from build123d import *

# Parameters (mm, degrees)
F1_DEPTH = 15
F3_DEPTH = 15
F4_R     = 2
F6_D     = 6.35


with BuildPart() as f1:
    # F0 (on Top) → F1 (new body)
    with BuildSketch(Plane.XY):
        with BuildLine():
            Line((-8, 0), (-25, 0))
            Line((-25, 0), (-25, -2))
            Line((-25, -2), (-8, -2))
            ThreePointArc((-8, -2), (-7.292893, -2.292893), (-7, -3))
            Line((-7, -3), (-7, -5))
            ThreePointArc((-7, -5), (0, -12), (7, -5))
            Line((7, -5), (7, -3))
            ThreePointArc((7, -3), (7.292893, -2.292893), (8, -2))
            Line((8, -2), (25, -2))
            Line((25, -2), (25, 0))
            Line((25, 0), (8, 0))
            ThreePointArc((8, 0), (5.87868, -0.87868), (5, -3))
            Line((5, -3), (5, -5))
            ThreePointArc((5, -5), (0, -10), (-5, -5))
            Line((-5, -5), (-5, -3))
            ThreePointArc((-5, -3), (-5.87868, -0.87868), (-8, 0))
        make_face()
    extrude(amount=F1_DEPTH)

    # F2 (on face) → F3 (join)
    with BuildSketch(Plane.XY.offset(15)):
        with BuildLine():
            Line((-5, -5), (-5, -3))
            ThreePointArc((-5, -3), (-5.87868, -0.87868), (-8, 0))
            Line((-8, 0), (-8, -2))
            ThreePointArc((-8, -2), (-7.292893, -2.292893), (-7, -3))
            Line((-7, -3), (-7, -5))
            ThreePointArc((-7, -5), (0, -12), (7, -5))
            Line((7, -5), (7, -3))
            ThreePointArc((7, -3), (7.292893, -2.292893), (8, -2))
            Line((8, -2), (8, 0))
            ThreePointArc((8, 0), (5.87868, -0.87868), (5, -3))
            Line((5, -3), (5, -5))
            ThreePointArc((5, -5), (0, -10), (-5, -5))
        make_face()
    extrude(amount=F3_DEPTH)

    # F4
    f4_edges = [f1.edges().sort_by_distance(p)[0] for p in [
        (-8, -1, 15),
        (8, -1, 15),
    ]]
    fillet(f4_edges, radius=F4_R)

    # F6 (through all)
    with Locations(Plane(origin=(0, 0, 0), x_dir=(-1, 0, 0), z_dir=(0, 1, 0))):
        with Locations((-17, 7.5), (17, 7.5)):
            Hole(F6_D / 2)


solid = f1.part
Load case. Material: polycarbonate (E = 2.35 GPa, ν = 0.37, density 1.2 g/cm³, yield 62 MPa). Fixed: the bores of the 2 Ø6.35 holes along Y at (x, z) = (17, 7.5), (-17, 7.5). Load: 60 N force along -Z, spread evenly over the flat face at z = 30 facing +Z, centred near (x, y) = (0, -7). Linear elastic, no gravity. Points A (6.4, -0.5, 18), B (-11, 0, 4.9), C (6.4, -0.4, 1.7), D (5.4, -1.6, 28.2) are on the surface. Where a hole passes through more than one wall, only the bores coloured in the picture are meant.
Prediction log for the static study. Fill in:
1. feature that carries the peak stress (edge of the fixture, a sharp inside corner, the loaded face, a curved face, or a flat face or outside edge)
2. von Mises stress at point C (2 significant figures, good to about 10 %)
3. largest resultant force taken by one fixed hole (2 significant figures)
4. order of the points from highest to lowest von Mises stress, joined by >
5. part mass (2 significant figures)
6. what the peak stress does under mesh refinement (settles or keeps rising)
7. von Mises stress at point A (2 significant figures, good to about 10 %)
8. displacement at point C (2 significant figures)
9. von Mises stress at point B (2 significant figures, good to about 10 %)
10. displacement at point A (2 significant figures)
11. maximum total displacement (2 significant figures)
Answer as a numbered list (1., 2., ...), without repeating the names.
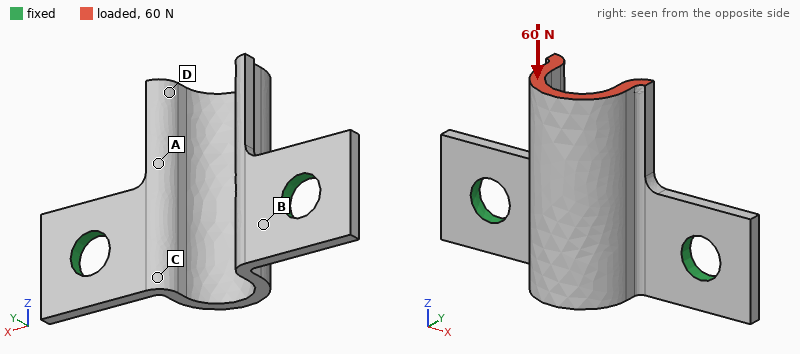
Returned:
1. edge of the fixture
2. 5.5 MPa
3. 30 N
4. B > C > A > D
5. 3.2 g
6. keeps rising
7. 2.7 MPa
8. 0.15 mm
9. 6.7 MPa
10. 0.26 mm
11. 0.65 mm
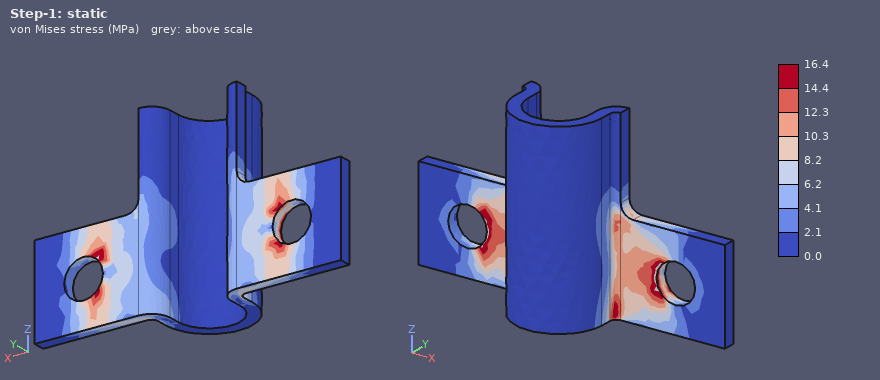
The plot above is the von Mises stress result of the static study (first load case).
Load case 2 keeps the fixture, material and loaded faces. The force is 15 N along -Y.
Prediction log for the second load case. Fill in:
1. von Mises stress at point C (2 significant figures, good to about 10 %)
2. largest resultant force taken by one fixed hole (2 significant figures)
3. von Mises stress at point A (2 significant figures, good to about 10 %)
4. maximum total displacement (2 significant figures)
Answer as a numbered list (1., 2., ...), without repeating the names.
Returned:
1. 4.9 MPa
2. 9.2 N
3. 3.2 MPa
4. 0.65 mm
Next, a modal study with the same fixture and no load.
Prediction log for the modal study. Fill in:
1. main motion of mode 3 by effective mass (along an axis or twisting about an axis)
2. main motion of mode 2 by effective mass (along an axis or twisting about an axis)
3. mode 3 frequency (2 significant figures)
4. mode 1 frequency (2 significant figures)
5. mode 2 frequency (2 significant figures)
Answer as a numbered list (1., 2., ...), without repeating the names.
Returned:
1. along X
2. along X
3. 3100 Hz
4. 950 Hz
5. 2300 Hz
